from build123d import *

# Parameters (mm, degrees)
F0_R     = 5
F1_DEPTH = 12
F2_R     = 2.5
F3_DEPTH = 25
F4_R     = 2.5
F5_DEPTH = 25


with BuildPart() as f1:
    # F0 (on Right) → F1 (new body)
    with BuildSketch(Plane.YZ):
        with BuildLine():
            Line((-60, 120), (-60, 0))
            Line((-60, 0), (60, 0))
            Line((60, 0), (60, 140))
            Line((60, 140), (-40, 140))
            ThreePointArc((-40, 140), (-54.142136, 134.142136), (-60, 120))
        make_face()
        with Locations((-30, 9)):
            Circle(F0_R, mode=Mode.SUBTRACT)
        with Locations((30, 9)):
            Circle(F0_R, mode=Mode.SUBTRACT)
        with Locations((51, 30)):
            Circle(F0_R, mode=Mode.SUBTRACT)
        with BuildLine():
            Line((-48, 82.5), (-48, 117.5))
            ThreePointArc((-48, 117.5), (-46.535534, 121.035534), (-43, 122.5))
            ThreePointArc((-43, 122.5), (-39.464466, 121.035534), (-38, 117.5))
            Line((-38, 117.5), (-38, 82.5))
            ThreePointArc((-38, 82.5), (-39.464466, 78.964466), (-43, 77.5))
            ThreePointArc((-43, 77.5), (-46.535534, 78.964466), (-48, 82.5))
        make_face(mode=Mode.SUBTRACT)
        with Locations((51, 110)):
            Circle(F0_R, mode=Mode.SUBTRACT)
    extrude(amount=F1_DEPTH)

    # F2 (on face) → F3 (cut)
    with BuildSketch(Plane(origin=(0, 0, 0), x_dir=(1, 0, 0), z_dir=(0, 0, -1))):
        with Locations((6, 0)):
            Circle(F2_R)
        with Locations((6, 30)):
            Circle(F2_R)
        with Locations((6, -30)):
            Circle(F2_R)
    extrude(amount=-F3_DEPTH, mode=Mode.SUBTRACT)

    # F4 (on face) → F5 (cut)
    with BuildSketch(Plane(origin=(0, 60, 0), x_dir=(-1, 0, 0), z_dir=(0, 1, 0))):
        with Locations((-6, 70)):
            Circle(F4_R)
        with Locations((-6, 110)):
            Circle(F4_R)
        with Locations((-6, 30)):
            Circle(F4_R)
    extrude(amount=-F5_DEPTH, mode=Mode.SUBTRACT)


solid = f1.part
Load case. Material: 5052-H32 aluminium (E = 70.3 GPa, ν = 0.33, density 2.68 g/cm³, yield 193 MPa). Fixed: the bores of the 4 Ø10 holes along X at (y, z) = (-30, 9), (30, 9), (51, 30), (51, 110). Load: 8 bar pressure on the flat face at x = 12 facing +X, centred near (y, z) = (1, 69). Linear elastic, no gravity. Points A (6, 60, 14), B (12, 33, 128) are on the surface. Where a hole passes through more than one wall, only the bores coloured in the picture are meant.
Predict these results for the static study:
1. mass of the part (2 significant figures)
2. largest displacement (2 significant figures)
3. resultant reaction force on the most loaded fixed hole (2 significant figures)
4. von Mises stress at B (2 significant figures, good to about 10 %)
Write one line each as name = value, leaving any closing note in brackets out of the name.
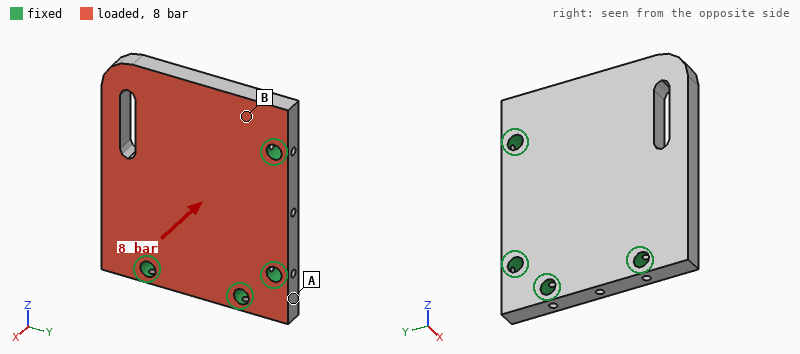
mass of the part = 510 g
largest displacement = 0.70 mm
resultant reaction force on the most loaded fixed hole = 5.7 kN
von Mises stress at B = 54 MPa
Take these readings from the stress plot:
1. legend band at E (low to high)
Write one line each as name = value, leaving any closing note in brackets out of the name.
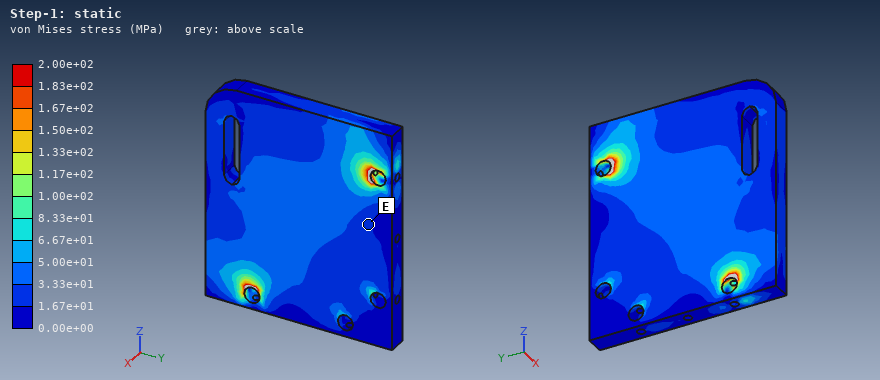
legend band at E = 1.67e+01 to 3.33e+01 MPa
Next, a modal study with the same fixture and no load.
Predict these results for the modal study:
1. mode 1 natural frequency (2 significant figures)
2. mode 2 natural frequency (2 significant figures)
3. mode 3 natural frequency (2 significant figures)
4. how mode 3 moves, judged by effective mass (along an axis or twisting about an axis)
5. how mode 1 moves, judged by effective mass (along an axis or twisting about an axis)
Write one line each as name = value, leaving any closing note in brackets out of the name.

mode 1 natural frequency = 1300 Hz
mode 2 natural frequency = 3800 Hz
mode 3 natural frequency = 4800 Hz
how mode 3 moves, judged by effective mass = along X
how mode 1 moves, judged by effective mass = along X
